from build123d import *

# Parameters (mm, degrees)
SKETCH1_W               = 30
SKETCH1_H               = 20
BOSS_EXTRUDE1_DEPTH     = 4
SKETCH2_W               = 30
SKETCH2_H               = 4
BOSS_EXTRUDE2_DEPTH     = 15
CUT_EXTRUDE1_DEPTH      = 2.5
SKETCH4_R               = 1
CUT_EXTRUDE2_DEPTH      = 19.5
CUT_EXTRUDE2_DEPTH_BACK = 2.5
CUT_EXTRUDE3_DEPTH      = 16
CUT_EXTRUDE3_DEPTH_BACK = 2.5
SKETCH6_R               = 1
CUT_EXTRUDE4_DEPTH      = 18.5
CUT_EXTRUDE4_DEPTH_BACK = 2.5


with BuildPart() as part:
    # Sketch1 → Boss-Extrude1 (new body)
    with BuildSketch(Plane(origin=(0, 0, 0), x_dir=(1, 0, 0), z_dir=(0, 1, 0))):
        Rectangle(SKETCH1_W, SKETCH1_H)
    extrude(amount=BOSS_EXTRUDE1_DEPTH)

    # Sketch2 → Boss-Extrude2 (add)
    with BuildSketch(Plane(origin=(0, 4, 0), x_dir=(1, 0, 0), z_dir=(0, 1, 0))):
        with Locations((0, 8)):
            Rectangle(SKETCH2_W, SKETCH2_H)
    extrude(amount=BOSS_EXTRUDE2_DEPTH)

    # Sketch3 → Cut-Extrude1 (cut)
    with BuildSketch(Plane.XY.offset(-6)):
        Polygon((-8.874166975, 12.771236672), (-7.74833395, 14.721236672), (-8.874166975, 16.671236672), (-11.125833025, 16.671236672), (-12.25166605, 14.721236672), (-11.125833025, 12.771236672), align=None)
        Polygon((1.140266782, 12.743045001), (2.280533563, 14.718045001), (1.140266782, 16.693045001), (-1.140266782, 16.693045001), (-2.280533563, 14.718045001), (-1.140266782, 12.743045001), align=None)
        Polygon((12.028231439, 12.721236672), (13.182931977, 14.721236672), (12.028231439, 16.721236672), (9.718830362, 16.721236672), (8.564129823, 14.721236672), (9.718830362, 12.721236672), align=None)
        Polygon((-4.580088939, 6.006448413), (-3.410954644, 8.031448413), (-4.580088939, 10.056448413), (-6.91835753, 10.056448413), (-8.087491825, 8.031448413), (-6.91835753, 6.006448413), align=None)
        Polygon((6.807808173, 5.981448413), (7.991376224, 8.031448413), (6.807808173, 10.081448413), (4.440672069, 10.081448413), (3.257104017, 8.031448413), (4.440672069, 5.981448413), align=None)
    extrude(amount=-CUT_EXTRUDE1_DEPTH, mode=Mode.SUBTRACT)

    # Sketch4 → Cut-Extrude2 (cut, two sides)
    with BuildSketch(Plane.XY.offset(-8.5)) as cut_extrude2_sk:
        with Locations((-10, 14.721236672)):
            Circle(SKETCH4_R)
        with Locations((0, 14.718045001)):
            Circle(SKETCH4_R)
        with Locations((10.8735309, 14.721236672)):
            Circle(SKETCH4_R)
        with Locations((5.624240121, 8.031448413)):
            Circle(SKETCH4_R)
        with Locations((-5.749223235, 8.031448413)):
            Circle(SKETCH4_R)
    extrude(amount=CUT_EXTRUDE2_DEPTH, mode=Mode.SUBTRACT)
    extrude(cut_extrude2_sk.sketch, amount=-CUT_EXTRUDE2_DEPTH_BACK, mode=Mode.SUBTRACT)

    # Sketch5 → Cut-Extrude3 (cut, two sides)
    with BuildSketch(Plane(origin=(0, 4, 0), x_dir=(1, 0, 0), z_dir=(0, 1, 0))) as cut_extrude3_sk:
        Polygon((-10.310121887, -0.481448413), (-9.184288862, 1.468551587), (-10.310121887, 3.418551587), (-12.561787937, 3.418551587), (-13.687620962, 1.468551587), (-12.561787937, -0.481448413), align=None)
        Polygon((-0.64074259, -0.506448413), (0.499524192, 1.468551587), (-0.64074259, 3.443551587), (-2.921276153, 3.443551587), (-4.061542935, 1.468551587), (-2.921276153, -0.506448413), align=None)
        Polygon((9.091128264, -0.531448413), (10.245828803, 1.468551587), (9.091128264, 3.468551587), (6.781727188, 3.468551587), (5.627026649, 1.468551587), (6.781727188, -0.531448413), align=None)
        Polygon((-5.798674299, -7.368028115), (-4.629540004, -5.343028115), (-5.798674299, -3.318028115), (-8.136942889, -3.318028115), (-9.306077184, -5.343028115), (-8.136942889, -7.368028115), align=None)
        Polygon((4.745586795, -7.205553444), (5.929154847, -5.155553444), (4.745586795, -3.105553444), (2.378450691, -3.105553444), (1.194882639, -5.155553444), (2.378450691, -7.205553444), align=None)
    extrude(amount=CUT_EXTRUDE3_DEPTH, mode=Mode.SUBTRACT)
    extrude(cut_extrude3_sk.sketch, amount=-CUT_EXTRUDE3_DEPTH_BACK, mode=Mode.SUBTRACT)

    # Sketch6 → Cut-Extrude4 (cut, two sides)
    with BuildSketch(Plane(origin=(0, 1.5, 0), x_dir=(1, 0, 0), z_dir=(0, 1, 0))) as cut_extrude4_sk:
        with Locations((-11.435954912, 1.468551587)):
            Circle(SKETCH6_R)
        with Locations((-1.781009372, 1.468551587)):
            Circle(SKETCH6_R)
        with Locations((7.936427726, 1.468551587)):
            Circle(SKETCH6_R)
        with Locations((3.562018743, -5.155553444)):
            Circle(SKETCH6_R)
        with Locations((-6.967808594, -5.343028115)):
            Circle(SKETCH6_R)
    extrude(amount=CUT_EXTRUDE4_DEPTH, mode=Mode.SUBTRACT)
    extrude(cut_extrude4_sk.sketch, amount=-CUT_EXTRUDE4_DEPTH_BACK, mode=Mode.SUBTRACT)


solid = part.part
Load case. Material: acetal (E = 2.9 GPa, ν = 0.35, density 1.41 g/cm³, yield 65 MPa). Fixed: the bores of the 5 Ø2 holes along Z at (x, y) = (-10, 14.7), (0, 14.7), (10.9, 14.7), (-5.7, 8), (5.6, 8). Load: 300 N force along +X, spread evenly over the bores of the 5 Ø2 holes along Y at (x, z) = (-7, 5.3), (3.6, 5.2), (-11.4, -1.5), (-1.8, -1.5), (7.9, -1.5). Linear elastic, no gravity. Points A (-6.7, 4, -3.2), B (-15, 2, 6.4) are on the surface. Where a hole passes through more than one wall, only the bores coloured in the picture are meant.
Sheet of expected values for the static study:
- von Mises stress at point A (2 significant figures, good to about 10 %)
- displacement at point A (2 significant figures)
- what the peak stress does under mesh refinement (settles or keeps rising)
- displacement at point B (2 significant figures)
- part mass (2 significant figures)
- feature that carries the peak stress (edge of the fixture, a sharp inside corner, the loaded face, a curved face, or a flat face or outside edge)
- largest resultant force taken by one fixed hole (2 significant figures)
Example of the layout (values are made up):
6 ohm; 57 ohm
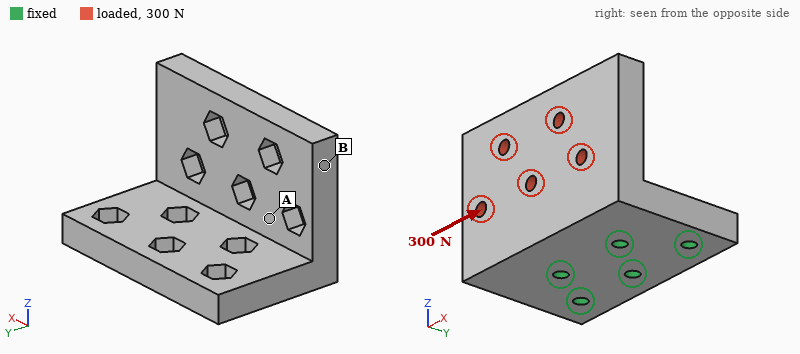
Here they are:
12 MPa; 0.16 mm; keeps rising; 0.39 mm; 5.4 g; edge of the fixture; 220 N
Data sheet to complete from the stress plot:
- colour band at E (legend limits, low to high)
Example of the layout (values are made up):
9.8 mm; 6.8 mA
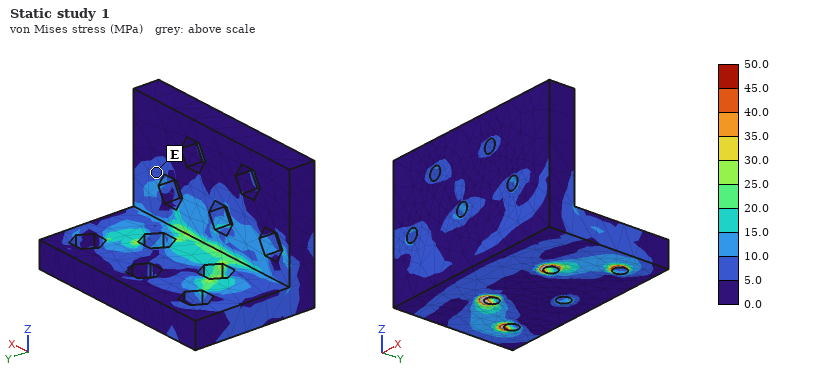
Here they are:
5.0 to 10.0 MPa
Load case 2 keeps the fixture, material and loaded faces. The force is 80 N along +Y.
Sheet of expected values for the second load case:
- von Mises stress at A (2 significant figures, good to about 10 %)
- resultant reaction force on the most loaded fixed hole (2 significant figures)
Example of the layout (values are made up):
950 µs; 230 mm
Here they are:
5.3 MPa; 55 N
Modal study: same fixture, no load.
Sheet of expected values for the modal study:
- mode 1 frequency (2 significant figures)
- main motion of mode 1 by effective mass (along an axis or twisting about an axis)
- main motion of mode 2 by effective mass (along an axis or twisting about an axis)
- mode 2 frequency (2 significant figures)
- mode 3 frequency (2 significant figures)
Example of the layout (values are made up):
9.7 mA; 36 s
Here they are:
1600 Hz; along Y; along X; 2400 Hz; 4000 Hz
